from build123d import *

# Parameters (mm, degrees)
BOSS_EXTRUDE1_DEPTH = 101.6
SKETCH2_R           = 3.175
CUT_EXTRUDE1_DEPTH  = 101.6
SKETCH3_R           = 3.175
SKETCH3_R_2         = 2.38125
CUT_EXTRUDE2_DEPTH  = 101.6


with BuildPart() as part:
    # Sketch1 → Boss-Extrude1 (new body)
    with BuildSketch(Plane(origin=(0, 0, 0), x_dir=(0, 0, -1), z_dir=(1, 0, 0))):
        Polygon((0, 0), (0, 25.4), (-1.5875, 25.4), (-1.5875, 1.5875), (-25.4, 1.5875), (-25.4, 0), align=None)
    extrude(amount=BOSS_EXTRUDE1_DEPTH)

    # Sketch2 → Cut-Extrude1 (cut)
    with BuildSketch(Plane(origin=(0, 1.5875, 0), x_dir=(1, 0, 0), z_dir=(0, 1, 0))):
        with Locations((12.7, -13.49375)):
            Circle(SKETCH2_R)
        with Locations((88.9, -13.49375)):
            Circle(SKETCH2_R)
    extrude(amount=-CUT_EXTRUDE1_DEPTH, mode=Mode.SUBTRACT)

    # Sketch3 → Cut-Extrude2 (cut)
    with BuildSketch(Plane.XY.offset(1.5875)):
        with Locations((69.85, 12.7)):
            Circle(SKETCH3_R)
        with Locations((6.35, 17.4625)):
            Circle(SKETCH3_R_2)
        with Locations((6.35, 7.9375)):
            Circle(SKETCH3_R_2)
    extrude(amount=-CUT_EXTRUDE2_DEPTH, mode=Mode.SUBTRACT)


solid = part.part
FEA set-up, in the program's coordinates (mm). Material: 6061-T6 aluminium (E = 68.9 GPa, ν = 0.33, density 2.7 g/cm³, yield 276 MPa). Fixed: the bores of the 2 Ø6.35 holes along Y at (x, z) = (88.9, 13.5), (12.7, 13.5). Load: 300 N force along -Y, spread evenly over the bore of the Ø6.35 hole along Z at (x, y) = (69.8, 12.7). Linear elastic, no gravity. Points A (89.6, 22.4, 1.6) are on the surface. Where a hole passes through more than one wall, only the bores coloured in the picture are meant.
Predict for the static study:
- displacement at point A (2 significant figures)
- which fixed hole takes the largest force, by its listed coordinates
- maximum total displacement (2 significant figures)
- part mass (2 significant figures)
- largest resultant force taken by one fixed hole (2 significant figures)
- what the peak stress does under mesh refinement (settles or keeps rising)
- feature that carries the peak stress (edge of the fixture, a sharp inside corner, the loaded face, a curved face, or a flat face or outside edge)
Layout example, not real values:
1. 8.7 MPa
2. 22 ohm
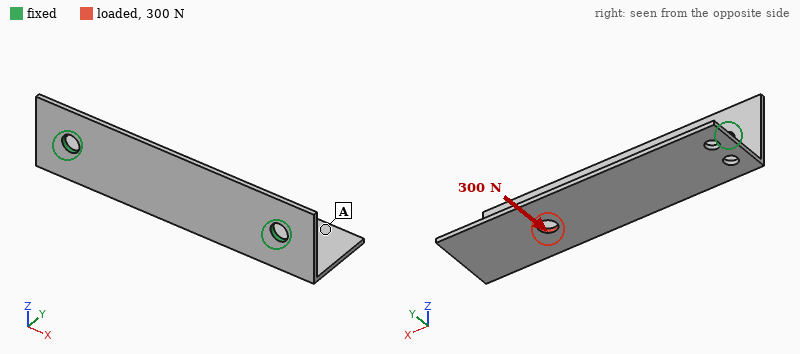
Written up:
1. 0.38 mm
2. (88.9, 13.5)
3. 0.46 mm
4. 21 g
5. 240 N
6. keeps rising
7. edge of the fixture
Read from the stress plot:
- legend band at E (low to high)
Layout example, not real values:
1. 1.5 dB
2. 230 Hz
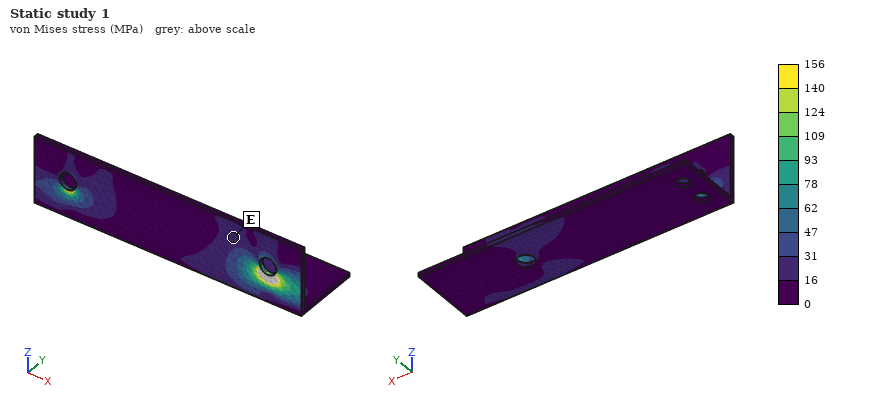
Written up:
1. 16 to 31 MPa
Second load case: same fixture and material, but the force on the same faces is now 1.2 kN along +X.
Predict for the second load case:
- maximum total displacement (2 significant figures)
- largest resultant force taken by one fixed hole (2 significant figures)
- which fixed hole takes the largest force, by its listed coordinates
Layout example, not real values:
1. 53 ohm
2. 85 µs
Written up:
1. 0.34 mm
2. 700 N
3. (88.9, 13.5)
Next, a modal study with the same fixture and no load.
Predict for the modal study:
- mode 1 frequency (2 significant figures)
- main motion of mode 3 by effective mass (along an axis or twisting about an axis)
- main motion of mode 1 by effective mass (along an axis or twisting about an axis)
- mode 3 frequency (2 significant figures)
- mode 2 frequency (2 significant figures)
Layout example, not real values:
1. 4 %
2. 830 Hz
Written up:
1. 1100 Hz
2. along Y
3. along Z
4. 2200 Hz
5. 1600 Hz
